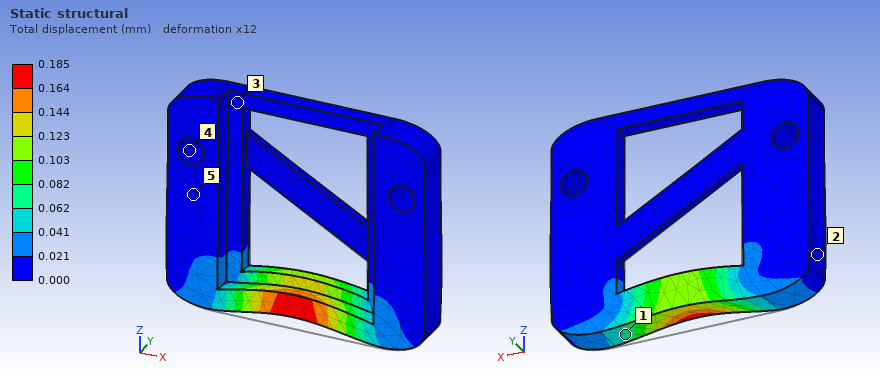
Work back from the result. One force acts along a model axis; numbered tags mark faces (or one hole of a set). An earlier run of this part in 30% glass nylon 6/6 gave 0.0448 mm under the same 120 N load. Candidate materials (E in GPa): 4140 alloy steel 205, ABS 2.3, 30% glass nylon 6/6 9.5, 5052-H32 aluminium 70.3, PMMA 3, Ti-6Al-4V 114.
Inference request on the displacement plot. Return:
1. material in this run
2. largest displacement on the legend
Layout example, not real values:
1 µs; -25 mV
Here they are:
ABS; 0.185 mm
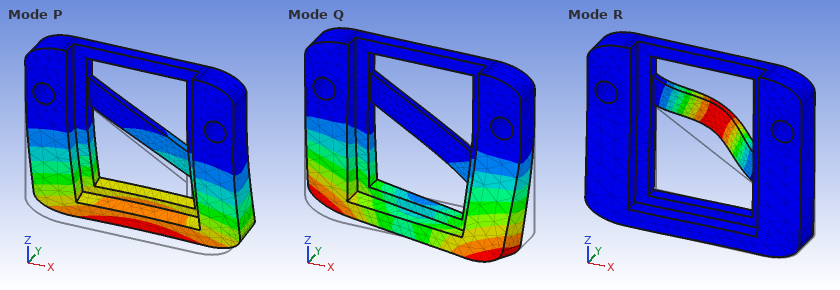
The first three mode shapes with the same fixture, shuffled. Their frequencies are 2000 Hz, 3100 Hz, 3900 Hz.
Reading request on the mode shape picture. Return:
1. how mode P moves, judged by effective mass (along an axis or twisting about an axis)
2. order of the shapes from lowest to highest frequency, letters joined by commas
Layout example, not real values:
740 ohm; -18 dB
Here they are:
along Y; P, Q, R
